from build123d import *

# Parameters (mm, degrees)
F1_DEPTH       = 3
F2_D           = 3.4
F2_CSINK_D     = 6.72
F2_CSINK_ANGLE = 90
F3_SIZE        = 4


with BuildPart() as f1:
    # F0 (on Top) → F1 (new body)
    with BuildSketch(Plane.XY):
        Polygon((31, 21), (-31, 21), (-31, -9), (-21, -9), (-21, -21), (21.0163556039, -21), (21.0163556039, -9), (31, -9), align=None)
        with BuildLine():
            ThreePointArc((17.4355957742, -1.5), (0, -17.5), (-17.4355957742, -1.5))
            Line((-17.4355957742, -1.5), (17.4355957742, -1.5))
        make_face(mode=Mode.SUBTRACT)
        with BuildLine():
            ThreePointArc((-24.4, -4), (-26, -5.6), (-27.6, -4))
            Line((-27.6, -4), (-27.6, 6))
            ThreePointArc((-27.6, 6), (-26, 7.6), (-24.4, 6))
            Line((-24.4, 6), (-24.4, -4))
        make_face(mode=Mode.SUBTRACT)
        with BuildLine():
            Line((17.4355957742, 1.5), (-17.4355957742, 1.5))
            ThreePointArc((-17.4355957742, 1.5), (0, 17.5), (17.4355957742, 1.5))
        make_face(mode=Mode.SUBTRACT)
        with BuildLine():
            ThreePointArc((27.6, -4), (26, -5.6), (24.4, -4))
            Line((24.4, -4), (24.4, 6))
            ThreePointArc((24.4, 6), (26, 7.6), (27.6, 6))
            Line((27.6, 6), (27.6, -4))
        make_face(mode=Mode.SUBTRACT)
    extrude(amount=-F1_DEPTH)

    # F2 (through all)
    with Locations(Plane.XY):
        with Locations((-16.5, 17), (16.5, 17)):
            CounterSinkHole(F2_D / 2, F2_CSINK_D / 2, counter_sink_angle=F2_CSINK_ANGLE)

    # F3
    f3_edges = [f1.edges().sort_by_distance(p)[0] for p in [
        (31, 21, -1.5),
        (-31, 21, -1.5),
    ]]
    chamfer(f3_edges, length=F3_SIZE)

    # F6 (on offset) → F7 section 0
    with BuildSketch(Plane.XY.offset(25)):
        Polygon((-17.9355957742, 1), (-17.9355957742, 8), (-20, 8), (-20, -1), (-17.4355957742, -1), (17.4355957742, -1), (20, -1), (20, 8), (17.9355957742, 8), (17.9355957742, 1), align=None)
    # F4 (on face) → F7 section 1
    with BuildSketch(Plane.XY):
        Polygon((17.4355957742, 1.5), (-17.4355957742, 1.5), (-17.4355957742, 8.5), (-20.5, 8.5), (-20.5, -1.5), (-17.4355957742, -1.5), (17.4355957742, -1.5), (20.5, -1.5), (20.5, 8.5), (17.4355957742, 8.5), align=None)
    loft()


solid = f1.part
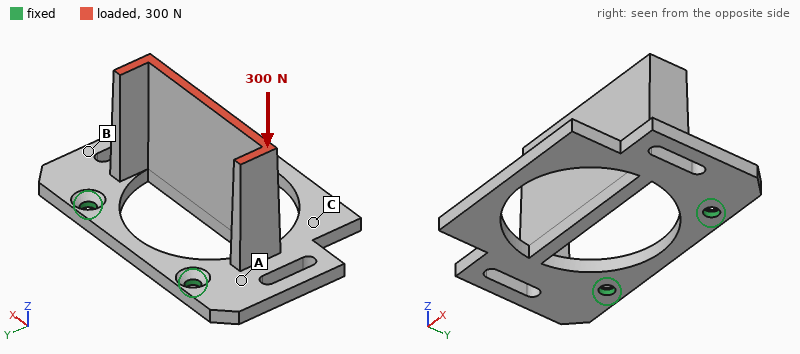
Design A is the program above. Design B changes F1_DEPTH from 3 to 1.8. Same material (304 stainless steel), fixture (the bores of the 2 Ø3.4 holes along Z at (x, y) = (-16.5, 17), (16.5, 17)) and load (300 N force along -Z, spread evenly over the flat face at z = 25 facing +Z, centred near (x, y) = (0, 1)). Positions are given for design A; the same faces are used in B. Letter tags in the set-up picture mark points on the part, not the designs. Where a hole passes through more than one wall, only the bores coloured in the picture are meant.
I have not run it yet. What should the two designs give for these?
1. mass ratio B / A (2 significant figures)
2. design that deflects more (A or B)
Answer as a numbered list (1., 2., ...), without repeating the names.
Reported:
1. 0.78
2. B
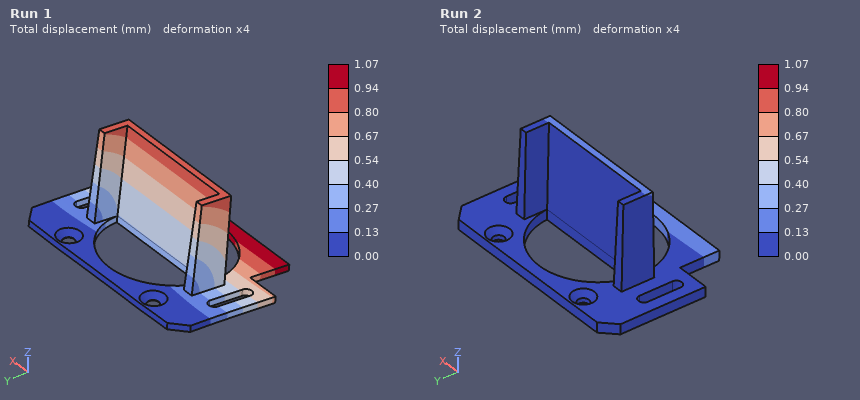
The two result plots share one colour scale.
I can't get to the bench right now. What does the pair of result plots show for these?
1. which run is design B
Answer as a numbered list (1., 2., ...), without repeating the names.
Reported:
1. Run 1
